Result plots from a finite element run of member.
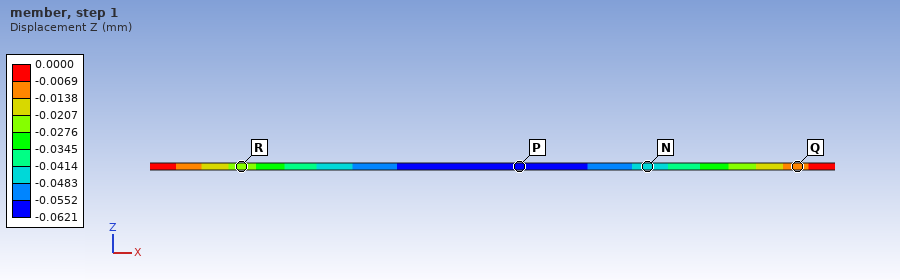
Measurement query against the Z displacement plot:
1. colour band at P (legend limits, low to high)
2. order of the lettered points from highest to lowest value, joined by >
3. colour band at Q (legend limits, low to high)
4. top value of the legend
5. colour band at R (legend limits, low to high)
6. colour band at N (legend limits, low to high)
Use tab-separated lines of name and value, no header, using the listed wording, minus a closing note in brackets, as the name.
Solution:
colour band at P	-0.0621 to -0.0552 mm
order of the lettered points from highest to lowest value, joined by >	Q > R > N > P
colour band at Q	-0.0138 to -0.0069 mm
top value of the legend	0.0000 mm
colour band at R	-0.0276 to -0.0207 mm
colour band at N	-0.0483 to -0.0414 mm
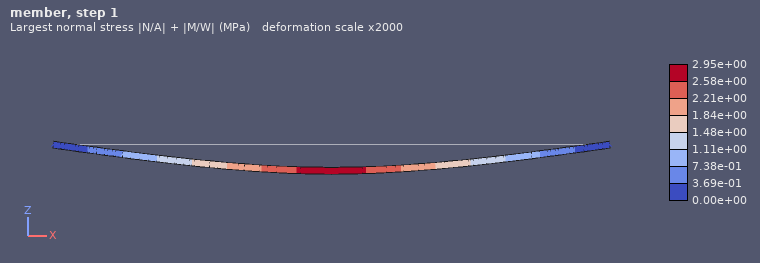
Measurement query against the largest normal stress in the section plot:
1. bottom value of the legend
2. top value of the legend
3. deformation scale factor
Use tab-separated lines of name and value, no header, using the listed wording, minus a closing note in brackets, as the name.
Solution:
bottom value of the legend	0.00e+00 MPa
top value of the legend	2.95e+00 MPa
deformation scale factor	2000
